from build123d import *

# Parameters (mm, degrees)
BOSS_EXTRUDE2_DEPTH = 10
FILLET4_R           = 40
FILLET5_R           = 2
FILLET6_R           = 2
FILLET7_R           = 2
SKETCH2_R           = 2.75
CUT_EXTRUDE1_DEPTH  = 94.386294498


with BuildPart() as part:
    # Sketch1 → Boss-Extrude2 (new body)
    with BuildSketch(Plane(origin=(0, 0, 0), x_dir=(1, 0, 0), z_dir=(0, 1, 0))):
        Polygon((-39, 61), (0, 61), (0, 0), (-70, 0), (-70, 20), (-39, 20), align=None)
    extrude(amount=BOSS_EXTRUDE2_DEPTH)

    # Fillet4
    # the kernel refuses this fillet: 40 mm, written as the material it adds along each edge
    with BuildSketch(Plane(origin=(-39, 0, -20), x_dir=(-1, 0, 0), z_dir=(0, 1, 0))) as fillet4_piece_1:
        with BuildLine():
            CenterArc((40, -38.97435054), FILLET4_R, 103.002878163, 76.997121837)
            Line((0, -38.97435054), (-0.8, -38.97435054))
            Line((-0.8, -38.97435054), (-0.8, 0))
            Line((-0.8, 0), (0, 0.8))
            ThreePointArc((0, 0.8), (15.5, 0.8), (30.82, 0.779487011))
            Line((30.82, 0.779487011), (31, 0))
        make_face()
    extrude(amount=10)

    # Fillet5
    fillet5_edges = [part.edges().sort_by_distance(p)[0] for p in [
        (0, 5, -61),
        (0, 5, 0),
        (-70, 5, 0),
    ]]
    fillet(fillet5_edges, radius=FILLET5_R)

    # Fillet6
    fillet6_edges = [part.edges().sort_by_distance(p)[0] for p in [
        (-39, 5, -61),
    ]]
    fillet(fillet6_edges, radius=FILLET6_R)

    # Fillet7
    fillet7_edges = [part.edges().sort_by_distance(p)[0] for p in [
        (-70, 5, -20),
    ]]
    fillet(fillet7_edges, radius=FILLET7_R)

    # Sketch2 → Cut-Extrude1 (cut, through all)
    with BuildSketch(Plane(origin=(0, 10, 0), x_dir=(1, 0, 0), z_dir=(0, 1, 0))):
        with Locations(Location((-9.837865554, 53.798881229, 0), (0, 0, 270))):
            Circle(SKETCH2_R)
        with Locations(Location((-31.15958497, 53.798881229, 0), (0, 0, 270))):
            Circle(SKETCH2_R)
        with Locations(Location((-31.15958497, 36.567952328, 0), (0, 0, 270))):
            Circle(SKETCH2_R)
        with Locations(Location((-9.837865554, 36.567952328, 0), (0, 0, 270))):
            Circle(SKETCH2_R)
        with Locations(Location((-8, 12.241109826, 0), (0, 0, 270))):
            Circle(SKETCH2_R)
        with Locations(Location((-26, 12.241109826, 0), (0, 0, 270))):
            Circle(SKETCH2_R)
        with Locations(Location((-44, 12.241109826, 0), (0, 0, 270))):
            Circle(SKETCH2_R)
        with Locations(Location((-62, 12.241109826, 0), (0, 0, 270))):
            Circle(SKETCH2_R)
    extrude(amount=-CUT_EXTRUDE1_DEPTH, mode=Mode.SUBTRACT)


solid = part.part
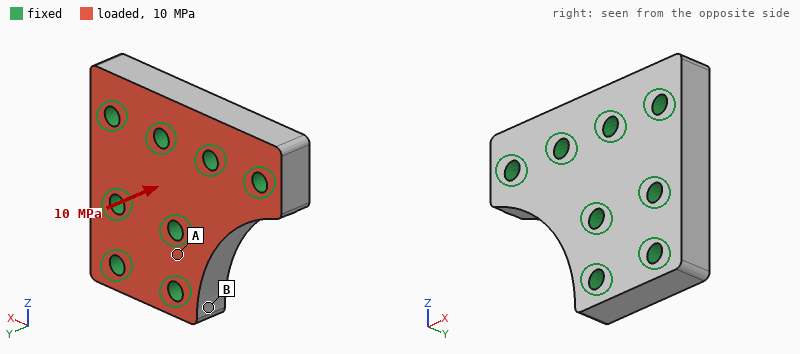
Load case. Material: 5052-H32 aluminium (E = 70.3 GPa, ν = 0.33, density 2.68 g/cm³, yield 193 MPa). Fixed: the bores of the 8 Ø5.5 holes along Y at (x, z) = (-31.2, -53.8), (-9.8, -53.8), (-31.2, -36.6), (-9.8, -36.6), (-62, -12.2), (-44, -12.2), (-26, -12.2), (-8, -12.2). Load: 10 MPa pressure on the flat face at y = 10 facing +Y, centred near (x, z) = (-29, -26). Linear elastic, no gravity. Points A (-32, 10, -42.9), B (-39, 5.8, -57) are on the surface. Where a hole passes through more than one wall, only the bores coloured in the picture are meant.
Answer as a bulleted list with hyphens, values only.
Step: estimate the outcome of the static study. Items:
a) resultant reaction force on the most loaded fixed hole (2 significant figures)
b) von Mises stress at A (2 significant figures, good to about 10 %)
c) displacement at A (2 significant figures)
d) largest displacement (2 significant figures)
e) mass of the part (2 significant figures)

- 4.7 kN
- 24 MPa
- 2.5 µm
- 13 µm
- 83 g
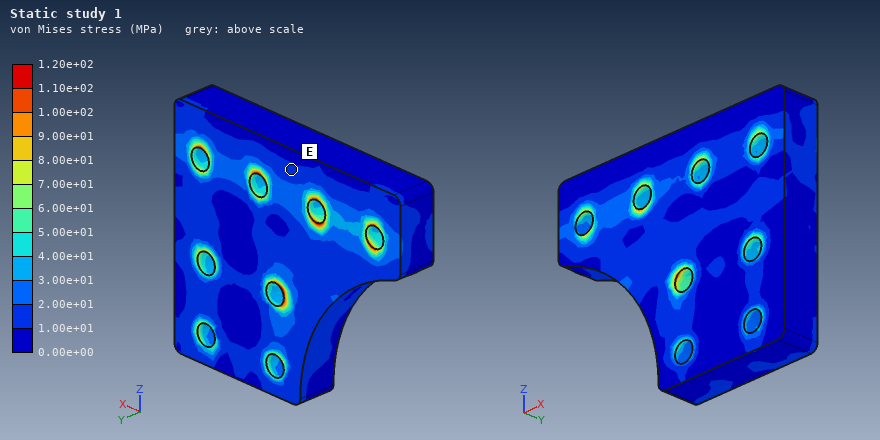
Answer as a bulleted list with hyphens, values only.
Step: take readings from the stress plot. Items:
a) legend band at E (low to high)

- 1.00e+01 to 2.00e+01 MPa
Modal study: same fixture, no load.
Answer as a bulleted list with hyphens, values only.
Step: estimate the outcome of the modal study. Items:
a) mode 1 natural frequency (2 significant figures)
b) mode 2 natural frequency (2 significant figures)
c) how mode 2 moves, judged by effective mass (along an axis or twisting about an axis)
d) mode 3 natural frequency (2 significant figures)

- 35 kHz
- 42 kHz
- along Y
- 44 kHz
